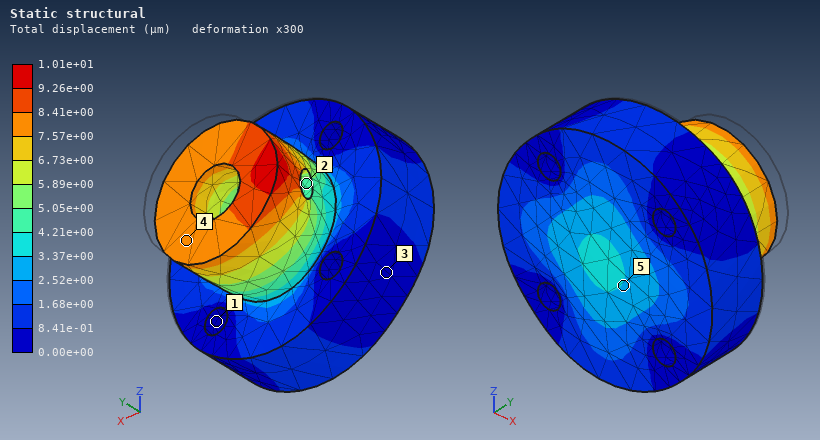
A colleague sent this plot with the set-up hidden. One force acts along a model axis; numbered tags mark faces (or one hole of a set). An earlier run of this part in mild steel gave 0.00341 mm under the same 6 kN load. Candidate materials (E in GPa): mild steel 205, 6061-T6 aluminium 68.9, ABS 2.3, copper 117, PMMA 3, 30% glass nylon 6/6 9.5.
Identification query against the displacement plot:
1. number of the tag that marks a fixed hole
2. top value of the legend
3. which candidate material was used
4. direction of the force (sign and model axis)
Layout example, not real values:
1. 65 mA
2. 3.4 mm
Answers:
1. 1
2. 1.01e+01 µm
3. 6061-T6 aluminium
4. -Y
